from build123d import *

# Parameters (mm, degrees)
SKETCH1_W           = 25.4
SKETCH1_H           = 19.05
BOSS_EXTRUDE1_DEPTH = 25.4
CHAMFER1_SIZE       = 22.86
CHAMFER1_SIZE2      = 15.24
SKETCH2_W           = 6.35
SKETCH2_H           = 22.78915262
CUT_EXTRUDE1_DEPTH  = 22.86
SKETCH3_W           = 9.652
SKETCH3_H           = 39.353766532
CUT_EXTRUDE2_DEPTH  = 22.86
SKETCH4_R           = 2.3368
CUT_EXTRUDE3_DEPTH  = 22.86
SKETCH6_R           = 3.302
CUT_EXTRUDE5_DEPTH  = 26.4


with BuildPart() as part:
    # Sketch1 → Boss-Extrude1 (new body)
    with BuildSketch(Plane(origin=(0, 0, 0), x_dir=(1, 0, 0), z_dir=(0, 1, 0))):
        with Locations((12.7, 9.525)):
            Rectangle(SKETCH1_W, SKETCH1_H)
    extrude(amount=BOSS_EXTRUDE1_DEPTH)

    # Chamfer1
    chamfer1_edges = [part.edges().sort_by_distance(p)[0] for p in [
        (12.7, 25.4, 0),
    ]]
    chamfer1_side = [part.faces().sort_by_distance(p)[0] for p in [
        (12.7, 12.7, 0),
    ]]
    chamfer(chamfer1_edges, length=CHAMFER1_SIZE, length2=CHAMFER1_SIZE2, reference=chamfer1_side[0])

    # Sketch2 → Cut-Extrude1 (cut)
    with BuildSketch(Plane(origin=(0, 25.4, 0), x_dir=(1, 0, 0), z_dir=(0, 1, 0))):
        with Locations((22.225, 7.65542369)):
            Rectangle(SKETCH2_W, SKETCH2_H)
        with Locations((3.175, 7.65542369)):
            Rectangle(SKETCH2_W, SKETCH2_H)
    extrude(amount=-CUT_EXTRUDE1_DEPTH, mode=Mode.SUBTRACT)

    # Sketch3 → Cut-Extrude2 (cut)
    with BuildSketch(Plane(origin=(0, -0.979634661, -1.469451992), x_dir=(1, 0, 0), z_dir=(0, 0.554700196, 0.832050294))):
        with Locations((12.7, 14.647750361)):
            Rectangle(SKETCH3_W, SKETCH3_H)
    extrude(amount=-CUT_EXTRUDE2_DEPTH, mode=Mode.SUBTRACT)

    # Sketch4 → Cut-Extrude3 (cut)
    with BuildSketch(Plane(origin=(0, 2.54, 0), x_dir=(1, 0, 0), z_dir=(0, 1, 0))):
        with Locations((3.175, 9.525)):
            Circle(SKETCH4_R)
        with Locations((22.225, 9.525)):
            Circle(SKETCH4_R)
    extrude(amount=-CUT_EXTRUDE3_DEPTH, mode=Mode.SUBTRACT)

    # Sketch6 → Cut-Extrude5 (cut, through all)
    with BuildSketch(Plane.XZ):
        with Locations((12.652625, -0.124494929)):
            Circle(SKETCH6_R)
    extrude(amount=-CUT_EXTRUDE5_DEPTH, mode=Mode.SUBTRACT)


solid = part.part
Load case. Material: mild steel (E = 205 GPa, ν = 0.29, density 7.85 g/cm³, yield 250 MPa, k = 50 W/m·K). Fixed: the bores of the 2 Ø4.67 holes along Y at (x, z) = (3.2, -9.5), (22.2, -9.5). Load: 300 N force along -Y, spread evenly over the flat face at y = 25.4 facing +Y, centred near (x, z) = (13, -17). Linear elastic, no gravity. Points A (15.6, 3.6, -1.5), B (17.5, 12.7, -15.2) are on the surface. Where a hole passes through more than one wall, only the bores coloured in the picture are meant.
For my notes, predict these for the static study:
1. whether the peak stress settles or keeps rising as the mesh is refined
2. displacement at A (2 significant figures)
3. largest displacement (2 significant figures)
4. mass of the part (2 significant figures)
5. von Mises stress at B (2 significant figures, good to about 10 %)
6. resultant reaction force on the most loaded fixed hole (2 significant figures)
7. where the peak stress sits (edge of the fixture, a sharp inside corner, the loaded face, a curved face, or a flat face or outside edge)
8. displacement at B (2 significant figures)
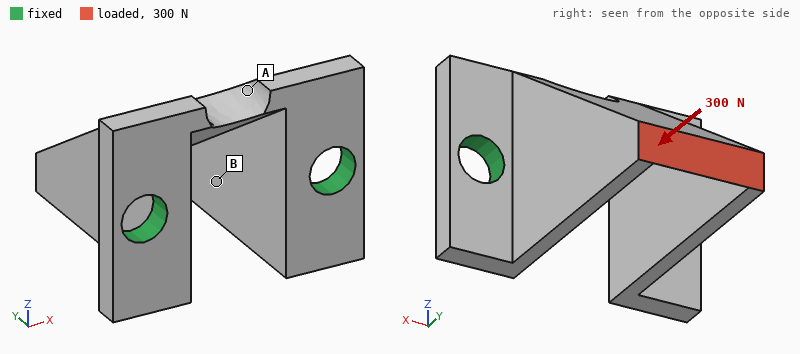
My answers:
keeps rising
2.6 µm
15 µm
18 g
16 MPa
150 N
edge of the fixture
5.7 µm
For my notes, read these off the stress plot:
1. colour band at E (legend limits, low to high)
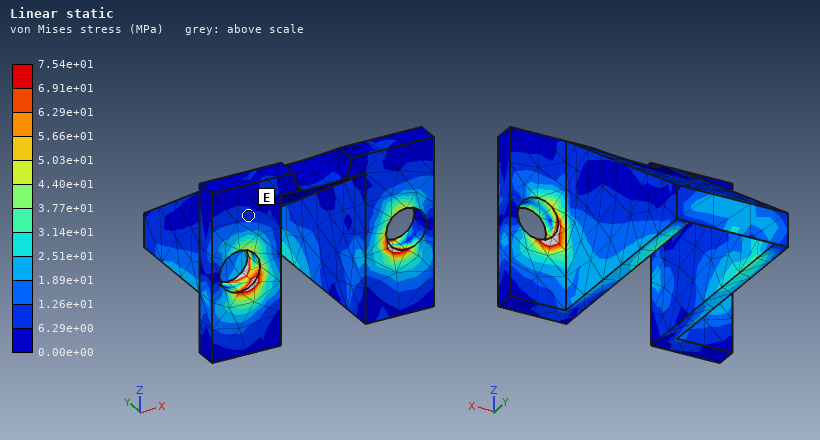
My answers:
6.29e+00 to 1.26e+01 MPa
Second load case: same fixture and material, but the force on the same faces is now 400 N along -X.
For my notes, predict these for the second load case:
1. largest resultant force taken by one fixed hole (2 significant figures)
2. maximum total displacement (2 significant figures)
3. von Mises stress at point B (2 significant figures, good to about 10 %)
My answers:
720 N
42 µm
53 MPa
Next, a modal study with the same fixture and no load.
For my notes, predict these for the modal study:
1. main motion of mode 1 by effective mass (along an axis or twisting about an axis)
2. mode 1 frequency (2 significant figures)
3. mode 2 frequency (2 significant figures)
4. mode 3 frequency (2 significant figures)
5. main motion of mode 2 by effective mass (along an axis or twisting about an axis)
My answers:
along Z
7200 Hz
8100 Hz
20 kHz
along X
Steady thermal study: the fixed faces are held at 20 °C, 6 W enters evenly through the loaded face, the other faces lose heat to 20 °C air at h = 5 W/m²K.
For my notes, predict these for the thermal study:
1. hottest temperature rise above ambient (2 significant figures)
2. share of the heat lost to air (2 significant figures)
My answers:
60 K
3.5 %
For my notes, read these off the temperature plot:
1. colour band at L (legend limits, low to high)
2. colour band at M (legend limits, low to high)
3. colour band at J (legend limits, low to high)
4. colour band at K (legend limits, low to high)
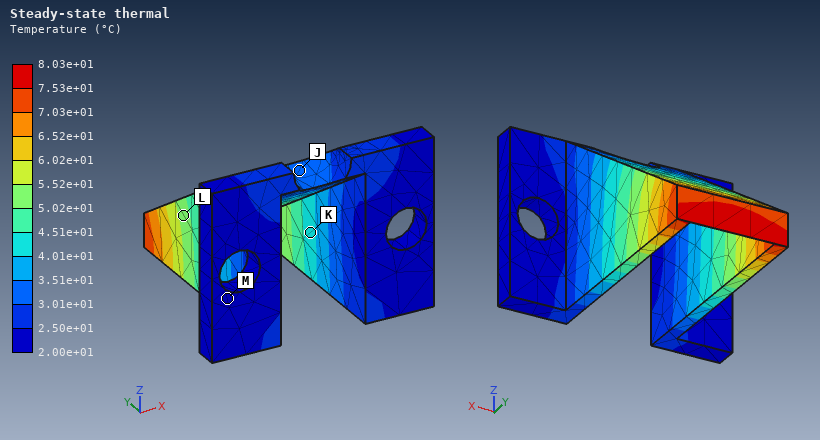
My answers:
5.02e+01 to 5.52e+01 °C
2.00e+01 to 2.50e+01 °C
3.01e+01 to 3.51e+01 °C
4.01e+01 to 4.51e+01 °C
